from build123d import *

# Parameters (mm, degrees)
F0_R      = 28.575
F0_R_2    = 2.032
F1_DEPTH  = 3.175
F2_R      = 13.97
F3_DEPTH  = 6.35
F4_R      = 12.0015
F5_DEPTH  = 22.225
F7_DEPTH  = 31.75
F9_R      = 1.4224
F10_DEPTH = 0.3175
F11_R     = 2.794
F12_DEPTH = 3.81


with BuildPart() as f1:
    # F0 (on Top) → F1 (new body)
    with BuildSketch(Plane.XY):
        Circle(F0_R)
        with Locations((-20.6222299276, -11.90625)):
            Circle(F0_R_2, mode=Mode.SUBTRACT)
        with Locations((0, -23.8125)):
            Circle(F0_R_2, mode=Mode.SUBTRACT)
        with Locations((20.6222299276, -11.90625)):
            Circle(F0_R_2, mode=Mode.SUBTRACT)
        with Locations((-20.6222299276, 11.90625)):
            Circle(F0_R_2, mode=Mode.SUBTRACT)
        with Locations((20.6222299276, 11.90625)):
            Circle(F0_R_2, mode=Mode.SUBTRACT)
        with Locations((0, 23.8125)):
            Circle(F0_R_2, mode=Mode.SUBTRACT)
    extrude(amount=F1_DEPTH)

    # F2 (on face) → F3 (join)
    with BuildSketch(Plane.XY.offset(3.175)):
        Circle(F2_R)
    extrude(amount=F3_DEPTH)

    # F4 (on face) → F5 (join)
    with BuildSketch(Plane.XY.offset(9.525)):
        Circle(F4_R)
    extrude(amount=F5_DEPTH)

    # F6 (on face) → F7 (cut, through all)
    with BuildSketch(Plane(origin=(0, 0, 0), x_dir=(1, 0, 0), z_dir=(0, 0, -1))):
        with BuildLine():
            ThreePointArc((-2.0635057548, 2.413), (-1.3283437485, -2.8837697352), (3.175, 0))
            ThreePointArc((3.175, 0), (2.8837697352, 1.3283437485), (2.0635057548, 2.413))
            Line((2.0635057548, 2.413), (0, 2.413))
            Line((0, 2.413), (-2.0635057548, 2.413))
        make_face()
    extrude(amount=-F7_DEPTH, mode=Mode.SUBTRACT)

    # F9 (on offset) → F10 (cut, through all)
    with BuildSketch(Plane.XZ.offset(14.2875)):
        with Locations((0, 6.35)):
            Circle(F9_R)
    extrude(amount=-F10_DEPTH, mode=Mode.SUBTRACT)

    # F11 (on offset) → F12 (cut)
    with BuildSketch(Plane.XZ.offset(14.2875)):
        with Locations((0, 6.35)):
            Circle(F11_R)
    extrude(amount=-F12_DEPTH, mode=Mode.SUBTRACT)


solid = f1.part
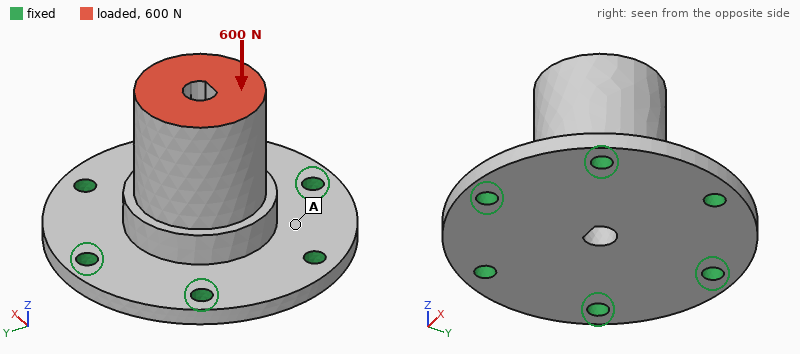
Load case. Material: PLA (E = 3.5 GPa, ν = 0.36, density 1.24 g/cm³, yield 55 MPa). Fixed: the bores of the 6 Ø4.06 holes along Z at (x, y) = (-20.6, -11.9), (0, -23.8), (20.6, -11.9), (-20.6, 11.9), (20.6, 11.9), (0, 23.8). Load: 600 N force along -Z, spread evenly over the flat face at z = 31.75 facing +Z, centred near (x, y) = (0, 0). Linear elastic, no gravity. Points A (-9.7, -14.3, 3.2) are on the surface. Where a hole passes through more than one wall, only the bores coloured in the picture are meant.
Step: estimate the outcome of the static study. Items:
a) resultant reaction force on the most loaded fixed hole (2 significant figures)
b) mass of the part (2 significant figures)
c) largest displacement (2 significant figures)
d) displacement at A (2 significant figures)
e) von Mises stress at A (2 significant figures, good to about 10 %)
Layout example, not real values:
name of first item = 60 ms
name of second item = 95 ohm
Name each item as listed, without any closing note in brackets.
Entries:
resultant reaction force on the most loaded fixed hole = 110 N
mass of the part = 26 g
largest displacement = 0.11 mm
displacement at A = 0.062 mm
von Mises stress at A = 5.3 MPa
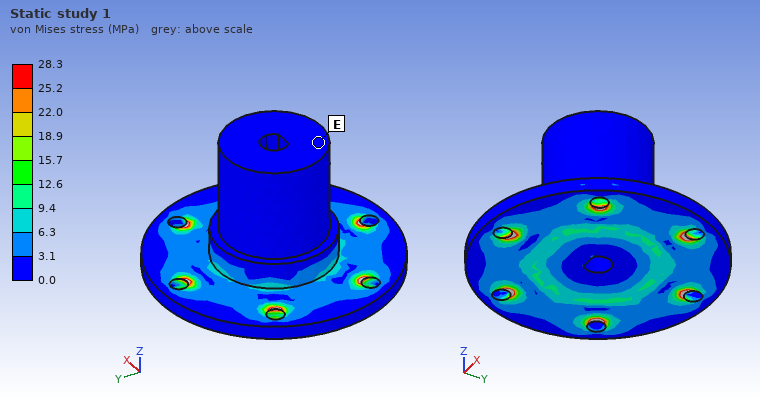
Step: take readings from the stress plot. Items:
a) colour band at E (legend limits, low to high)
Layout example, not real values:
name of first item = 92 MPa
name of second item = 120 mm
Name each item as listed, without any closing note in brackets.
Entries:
colour band at E = 0.0 to 3.1 MPa
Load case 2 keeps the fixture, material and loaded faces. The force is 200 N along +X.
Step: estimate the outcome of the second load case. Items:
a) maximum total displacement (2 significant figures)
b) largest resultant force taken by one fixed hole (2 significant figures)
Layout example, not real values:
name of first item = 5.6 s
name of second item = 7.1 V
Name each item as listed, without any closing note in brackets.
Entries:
maximum total displacement = 0.20 mm
largest resultant force taken by one fixed hole = 100 N
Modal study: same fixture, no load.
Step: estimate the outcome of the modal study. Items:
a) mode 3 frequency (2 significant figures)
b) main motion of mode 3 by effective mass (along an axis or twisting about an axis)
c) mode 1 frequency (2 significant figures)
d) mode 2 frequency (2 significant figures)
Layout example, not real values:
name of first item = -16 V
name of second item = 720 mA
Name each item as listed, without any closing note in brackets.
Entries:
mode 3 frequency = 2800 Hz
main motion of mode 3 by effective mass = along Z
mode 1 frequency = 2100 Hz
mode 2 frequency = 2200 Hz
